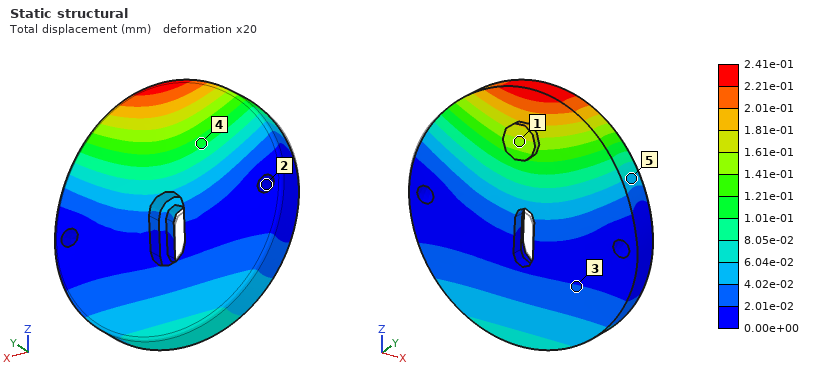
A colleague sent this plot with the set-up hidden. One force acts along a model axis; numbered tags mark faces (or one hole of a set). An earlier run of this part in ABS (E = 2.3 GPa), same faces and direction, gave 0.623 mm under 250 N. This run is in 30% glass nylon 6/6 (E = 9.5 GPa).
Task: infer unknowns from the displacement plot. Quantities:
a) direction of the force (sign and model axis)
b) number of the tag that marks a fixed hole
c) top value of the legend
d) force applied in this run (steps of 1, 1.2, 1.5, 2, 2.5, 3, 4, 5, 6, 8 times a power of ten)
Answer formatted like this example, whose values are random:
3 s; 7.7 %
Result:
+Y; 2; 2.41e-01 mm; 400 N
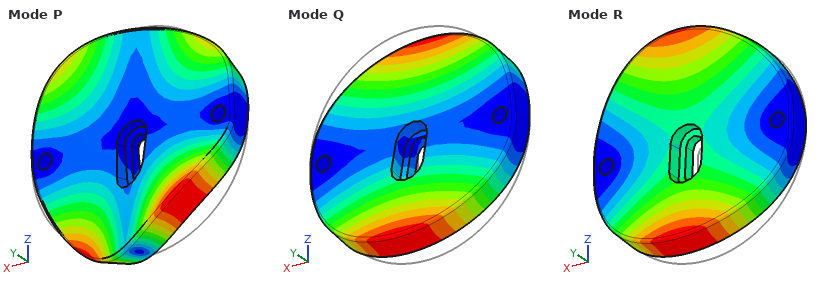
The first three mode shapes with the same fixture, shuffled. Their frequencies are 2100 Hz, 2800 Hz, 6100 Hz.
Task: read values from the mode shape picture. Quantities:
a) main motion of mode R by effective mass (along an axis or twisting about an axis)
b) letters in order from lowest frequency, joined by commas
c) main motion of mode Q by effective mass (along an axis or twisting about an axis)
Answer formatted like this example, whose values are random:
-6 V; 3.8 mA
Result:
along Y; Q, R, P; twisting about X
